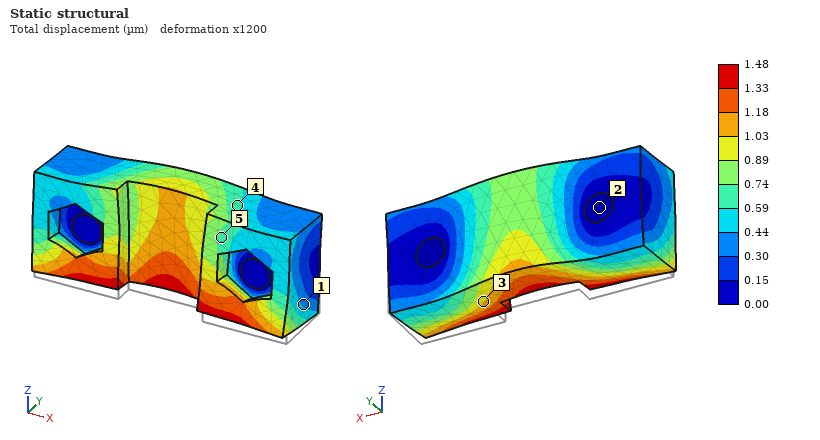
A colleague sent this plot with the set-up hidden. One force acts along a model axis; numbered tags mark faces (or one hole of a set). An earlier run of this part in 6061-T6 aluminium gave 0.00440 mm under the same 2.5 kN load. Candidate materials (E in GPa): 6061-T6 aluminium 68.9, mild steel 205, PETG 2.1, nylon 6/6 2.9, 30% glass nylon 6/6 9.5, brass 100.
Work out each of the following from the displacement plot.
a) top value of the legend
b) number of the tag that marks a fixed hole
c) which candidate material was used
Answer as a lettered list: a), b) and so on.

a) 1.48 µm
b) 2
c) mild steel
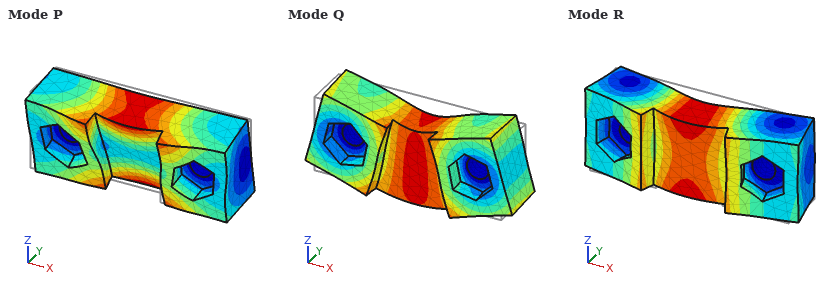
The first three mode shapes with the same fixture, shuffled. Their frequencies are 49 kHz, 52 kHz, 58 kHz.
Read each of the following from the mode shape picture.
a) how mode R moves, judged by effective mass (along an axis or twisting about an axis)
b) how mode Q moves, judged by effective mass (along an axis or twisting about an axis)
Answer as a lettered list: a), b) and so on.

a) along Y
b) along Z
